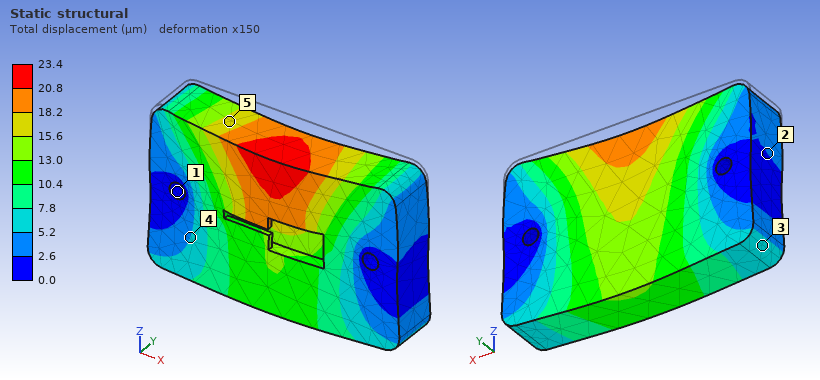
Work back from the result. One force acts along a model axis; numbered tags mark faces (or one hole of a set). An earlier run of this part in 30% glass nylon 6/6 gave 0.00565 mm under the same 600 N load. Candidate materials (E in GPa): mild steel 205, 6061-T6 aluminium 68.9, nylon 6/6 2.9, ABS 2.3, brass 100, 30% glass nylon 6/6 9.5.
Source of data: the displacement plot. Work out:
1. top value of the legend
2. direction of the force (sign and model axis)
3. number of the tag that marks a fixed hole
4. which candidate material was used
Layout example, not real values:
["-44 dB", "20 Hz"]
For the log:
["23.4 µm", "-Z", "1", "ABS"]
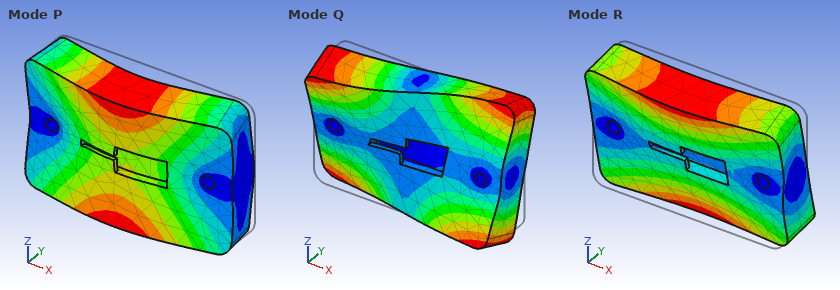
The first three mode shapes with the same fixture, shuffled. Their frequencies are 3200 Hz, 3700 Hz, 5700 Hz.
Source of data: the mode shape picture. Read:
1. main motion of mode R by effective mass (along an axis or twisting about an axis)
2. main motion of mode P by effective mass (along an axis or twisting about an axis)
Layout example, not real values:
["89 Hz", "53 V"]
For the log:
["twisting about X", "along Y"]
